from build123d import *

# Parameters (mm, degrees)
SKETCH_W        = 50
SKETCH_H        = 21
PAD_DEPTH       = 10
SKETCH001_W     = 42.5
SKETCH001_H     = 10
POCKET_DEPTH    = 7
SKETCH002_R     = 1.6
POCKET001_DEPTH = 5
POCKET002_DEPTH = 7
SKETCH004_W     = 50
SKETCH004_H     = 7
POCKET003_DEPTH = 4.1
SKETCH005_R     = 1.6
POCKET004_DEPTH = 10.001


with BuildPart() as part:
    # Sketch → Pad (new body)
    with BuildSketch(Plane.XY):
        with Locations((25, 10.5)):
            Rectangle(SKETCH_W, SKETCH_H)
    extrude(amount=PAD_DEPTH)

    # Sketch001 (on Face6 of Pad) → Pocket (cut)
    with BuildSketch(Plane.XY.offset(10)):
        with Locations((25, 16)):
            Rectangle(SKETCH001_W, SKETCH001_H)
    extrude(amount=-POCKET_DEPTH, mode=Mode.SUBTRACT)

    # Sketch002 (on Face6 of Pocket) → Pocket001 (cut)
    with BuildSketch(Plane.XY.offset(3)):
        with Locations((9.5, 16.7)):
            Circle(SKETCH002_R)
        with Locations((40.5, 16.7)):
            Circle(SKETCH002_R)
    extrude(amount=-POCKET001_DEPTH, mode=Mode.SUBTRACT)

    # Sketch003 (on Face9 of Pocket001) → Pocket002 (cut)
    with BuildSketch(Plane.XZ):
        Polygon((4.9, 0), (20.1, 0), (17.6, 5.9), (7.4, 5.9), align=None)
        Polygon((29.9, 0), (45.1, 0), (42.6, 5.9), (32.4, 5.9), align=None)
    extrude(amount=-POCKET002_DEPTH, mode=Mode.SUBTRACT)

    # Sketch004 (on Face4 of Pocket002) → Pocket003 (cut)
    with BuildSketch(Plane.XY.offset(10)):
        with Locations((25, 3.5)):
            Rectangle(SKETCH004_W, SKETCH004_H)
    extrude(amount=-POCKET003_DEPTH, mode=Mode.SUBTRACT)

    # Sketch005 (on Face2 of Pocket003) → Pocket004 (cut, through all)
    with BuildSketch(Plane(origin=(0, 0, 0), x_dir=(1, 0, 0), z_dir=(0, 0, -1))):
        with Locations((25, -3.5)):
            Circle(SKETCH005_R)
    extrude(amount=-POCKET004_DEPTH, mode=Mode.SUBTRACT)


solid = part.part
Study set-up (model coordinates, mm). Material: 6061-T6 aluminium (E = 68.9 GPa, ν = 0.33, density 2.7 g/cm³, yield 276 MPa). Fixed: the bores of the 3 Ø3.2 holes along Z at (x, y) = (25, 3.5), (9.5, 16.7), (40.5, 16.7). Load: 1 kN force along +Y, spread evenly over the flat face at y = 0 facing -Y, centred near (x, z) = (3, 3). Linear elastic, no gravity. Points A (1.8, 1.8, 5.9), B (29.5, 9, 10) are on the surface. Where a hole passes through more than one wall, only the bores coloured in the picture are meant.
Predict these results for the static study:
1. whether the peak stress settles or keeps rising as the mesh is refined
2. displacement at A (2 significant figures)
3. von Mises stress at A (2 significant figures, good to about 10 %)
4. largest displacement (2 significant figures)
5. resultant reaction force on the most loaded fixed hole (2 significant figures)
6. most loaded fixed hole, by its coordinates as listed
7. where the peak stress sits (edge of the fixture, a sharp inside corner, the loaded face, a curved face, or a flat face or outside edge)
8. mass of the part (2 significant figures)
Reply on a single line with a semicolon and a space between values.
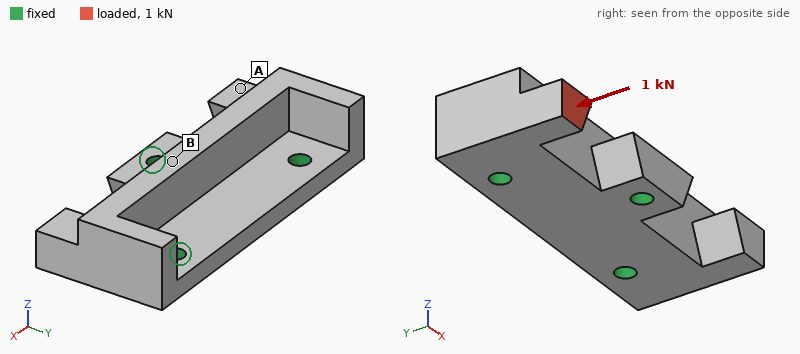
keeps rising; 36 µm; 27 MPa; 42 µm; 1.1 kN; (9.5, 16.7); edge of the fixture; 13 g
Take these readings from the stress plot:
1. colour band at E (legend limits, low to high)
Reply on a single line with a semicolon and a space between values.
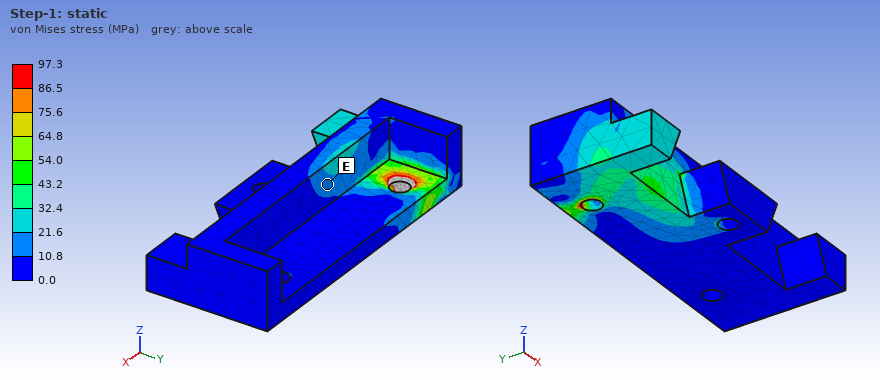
10.8 to 21.6 MPa
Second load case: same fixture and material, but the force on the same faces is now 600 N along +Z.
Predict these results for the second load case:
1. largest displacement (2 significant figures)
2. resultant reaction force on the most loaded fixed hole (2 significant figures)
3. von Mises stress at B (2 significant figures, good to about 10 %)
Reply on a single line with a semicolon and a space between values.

0.18 mm; 450 N; 28 MPa
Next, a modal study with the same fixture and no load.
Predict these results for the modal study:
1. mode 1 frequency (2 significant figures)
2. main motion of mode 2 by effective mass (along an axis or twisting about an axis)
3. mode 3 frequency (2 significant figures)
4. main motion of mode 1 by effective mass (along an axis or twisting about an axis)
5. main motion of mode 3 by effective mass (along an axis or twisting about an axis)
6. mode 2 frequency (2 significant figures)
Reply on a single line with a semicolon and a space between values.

10 kHz; along Z; 22 kHz; twisting about Y; along X; 11 kHz
